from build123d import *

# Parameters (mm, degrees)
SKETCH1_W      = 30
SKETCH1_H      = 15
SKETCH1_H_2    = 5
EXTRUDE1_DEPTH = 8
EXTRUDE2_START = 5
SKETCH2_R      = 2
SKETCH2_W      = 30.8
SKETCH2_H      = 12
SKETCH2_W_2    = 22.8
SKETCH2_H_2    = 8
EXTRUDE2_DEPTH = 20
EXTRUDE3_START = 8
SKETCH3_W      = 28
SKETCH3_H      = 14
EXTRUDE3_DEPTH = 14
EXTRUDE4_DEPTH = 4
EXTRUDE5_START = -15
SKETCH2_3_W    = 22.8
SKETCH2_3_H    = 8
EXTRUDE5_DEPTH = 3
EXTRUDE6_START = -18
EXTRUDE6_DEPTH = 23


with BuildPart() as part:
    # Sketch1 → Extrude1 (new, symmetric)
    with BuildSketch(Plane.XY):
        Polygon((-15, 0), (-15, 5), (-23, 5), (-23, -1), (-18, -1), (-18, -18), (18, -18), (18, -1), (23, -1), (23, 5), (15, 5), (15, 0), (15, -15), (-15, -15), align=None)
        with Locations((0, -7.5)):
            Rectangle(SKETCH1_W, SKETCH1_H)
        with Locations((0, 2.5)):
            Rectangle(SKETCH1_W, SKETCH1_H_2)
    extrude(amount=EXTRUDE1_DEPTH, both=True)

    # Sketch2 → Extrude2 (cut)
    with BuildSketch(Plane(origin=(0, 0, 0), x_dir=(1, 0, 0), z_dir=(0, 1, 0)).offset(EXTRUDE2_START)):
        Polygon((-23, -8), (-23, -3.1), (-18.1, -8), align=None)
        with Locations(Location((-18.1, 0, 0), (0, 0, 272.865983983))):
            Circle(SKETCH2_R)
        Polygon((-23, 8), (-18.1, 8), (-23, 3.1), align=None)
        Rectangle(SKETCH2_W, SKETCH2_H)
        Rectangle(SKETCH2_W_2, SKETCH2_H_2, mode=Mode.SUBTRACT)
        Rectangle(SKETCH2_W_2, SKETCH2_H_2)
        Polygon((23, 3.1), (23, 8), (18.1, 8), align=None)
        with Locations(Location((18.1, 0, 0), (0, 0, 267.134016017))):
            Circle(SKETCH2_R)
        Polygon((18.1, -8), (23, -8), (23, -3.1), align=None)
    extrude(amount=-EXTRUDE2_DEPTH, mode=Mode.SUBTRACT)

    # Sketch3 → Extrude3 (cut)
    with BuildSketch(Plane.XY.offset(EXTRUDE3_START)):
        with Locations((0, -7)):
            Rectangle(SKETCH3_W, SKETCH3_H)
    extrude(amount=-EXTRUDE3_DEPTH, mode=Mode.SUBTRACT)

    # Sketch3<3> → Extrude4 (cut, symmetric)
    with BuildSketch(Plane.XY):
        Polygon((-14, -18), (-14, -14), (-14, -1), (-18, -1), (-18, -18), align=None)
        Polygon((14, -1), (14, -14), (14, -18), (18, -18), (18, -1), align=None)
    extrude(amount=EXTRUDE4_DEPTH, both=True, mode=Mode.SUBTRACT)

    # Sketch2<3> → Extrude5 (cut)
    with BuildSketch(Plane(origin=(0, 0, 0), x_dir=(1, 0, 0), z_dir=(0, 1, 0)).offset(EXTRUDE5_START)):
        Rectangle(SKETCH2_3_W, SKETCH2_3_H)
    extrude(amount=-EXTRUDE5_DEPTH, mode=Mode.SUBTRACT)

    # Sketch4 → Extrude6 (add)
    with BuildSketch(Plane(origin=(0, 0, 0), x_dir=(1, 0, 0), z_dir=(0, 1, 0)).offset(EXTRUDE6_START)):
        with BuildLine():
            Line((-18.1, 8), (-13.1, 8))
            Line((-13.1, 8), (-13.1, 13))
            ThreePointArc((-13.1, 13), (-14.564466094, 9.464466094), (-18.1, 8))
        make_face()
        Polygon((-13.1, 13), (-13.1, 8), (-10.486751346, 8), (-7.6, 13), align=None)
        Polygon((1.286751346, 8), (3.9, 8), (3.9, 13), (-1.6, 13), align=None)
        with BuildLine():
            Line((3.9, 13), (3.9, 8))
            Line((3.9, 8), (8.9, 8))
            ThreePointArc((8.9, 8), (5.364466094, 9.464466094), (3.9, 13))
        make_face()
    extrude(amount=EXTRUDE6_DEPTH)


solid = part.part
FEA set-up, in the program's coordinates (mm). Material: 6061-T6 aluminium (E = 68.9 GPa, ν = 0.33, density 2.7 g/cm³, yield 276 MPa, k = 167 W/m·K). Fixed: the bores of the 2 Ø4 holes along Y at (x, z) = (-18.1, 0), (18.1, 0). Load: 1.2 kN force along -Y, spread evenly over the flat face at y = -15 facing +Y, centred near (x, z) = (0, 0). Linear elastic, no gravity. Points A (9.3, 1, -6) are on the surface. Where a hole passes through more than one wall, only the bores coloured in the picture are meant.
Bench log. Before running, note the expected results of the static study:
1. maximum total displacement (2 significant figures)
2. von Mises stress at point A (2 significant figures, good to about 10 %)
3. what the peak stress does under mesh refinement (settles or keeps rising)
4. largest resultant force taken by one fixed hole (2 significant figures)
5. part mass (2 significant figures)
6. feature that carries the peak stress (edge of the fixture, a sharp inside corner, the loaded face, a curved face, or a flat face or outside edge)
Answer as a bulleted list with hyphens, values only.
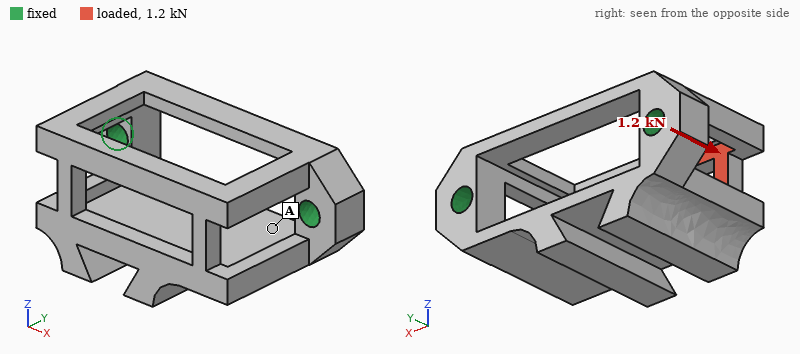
- 87 µm
- 19 MPa
- keeps rising
- 620 N
- 15 g
- a sharp inside corner
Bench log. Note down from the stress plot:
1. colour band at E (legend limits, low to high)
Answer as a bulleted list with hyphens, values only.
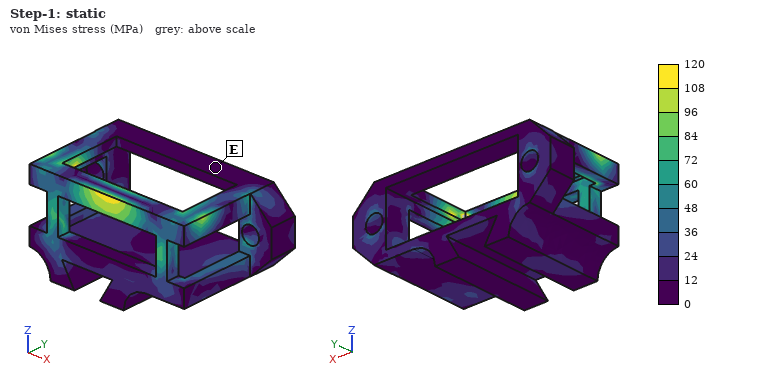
- 0 to 12 MPa
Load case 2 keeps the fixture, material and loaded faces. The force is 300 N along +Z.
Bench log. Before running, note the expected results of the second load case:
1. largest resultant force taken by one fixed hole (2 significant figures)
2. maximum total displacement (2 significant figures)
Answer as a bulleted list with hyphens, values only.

- 160 N
- 71 µm
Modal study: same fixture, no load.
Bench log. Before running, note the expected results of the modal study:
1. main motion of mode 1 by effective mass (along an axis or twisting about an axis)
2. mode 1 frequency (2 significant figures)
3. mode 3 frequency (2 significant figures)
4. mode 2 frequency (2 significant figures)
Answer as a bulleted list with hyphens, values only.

- along Z
- 4700 Hz
- 8500 Hz
- 7900 Hz
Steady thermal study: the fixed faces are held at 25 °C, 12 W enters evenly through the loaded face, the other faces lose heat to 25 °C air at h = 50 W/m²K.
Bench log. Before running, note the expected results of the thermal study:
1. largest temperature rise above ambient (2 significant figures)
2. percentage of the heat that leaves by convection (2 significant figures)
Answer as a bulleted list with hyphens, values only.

- 22 K
- 16 %
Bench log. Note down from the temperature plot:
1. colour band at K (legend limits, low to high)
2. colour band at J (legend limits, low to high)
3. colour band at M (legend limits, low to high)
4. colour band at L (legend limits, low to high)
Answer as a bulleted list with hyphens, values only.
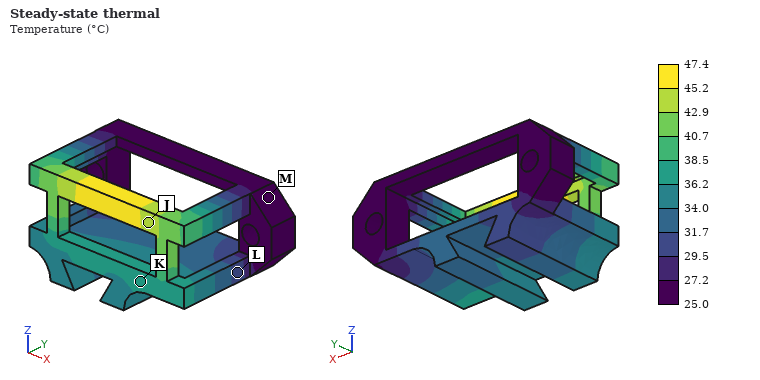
- 36.2 to 38.5 °C
- 42.9 to 45.2 °C
- 25.0 to 27.2 °C
- 29.5 to 31.7 °C
